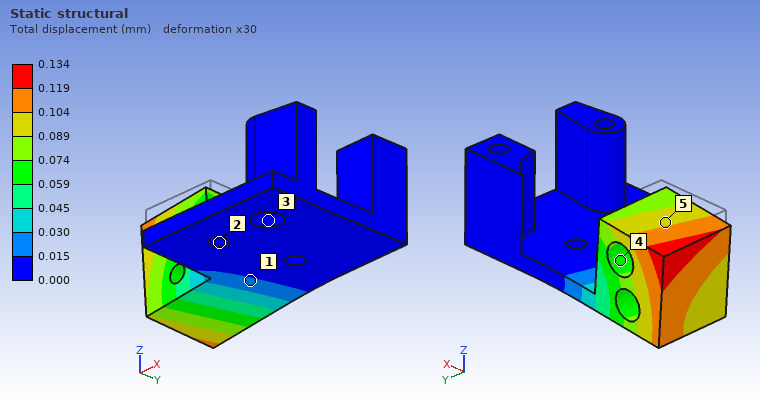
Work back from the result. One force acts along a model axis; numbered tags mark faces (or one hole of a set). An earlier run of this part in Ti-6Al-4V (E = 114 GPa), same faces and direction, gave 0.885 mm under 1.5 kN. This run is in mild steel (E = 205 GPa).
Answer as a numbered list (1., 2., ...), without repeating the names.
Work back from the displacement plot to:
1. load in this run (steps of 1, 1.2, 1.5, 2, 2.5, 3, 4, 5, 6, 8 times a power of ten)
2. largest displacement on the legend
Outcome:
1. 400 N
2. 0.134 mm
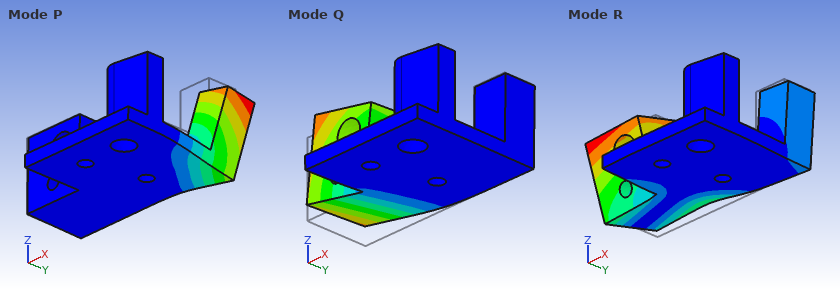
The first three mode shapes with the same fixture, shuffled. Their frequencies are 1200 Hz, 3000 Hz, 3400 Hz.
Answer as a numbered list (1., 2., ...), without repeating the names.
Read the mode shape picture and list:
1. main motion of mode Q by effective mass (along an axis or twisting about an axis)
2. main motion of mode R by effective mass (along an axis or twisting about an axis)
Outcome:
1. along Z
2. along Y
